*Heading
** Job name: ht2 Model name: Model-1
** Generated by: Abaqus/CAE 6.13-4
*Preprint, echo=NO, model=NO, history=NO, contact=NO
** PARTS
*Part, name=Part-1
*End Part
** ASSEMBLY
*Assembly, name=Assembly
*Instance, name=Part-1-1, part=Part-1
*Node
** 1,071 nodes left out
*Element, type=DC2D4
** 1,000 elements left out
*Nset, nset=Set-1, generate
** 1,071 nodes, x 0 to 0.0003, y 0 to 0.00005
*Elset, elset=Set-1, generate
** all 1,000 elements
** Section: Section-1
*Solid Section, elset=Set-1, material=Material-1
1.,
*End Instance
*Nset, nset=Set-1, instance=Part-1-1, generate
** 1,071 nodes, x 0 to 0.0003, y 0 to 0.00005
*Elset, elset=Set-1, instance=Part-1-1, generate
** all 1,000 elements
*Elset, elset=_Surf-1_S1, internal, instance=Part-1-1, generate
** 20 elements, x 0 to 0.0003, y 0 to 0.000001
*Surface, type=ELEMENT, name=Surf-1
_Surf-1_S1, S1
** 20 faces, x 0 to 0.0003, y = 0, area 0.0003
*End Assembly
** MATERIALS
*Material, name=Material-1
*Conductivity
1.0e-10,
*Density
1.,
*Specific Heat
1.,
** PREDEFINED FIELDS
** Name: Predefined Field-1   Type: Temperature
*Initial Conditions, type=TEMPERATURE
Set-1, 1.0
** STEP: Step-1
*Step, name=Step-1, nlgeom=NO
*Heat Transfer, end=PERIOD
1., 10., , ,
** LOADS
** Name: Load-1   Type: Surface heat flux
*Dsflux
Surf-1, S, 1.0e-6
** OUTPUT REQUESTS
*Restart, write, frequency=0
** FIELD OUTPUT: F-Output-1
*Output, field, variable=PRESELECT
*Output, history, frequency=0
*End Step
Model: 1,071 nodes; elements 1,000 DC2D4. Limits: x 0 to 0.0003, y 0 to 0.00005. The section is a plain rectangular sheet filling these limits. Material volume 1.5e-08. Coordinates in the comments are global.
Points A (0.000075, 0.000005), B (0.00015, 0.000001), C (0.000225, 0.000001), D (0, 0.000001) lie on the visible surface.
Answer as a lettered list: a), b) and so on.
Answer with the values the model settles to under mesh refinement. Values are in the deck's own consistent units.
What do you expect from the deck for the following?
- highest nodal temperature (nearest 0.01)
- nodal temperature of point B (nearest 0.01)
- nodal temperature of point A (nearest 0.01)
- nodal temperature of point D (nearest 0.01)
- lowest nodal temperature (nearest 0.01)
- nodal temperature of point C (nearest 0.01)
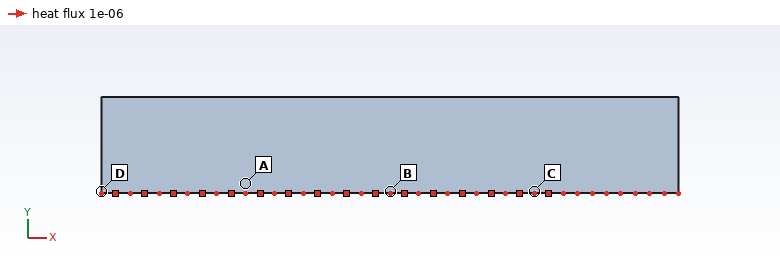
a) 1.36
b) 1.35
c) 1.32
d) 1.35
e) 1.12
f) 1.35
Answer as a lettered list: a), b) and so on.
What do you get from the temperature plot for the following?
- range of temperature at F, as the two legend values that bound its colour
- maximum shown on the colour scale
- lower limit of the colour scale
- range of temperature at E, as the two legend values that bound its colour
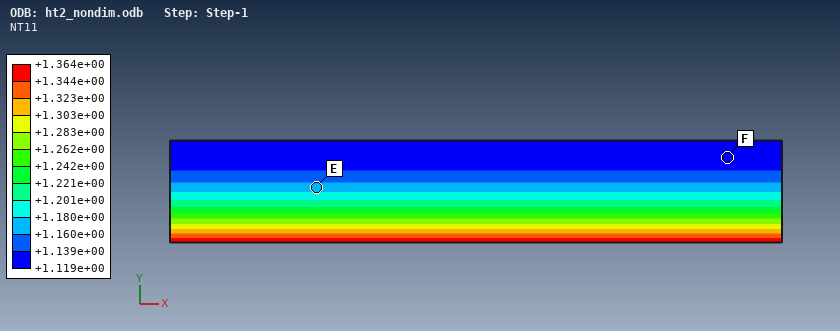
a) +1.119e+00 to +1.139e+00
b) +1.364e+00
c) +1.119e+00
d) +1.160e+00 to +1.180e+00
